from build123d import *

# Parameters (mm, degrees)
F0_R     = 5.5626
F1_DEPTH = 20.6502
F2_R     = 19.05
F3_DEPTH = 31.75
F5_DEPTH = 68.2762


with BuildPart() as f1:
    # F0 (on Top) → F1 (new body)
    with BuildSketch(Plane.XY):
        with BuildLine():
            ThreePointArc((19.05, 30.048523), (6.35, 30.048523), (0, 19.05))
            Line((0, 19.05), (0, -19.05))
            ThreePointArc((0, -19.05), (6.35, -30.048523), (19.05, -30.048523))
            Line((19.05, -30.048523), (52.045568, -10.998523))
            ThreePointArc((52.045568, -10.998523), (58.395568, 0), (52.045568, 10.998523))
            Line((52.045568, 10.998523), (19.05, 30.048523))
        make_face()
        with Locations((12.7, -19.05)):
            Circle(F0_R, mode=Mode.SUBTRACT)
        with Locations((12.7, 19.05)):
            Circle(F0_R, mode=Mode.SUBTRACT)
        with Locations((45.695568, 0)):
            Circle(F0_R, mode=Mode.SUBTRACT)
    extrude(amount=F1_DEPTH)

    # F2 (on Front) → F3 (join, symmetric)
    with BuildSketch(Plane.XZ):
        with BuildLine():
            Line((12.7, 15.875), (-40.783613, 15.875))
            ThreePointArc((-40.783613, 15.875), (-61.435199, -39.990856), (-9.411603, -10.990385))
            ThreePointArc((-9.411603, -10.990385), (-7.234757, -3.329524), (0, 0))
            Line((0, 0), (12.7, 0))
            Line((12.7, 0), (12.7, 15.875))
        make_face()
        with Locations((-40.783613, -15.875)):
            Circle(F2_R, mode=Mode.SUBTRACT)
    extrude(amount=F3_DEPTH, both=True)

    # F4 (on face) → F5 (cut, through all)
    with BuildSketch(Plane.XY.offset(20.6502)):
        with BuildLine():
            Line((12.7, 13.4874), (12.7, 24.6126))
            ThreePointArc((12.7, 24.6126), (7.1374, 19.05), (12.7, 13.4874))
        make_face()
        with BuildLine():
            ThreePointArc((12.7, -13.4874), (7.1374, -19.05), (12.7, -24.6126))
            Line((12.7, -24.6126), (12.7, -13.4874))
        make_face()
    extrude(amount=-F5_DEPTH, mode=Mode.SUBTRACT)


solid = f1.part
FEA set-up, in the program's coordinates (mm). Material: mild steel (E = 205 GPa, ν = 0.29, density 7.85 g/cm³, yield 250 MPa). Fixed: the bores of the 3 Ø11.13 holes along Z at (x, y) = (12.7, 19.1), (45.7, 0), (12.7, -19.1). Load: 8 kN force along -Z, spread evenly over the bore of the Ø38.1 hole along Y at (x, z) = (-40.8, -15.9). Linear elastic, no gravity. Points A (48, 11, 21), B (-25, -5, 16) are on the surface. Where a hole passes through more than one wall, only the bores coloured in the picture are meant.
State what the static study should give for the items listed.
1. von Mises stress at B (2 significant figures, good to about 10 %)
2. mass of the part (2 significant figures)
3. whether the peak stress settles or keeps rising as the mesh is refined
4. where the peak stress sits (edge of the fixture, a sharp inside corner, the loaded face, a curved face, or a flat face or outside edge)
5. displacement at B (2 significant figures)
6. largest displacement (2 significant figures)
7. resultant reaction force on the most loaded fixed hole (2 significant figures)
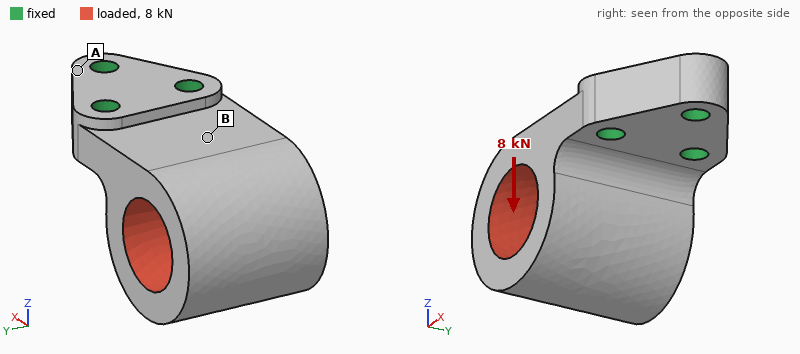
29 MPa
1.6 kg
keeps rising
edge of the fixture
0.037 mm
0.13 mm
4.7 kN
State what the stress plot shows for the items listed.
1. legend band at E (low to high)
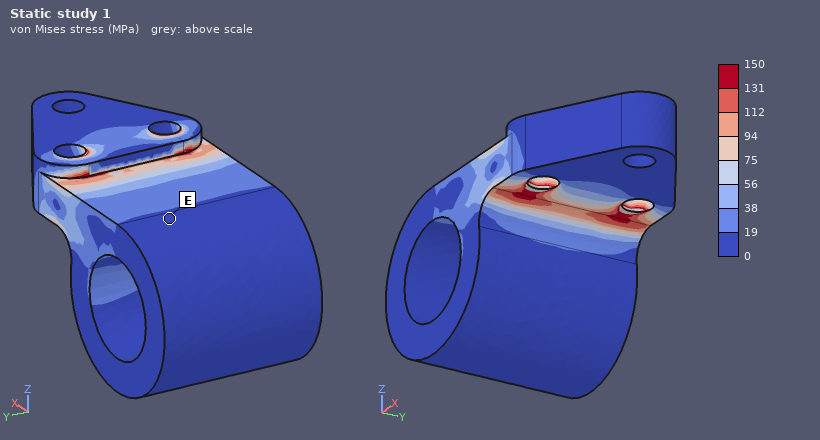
0 to 19 MPa
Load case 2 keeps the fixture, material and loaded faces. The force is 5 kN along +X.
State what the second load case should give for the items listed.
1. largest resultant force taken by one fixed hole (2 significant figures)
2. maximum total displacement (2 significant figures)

2.4 kN
49 µm
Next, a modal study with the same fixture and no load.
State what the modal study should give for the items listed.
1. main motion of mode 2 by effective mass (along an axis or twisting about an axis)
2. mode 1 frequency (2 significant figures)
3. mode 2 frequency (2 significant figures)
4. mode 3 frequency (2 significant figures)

along Y
1300 Hz
3100 Hz
5100 Hz
